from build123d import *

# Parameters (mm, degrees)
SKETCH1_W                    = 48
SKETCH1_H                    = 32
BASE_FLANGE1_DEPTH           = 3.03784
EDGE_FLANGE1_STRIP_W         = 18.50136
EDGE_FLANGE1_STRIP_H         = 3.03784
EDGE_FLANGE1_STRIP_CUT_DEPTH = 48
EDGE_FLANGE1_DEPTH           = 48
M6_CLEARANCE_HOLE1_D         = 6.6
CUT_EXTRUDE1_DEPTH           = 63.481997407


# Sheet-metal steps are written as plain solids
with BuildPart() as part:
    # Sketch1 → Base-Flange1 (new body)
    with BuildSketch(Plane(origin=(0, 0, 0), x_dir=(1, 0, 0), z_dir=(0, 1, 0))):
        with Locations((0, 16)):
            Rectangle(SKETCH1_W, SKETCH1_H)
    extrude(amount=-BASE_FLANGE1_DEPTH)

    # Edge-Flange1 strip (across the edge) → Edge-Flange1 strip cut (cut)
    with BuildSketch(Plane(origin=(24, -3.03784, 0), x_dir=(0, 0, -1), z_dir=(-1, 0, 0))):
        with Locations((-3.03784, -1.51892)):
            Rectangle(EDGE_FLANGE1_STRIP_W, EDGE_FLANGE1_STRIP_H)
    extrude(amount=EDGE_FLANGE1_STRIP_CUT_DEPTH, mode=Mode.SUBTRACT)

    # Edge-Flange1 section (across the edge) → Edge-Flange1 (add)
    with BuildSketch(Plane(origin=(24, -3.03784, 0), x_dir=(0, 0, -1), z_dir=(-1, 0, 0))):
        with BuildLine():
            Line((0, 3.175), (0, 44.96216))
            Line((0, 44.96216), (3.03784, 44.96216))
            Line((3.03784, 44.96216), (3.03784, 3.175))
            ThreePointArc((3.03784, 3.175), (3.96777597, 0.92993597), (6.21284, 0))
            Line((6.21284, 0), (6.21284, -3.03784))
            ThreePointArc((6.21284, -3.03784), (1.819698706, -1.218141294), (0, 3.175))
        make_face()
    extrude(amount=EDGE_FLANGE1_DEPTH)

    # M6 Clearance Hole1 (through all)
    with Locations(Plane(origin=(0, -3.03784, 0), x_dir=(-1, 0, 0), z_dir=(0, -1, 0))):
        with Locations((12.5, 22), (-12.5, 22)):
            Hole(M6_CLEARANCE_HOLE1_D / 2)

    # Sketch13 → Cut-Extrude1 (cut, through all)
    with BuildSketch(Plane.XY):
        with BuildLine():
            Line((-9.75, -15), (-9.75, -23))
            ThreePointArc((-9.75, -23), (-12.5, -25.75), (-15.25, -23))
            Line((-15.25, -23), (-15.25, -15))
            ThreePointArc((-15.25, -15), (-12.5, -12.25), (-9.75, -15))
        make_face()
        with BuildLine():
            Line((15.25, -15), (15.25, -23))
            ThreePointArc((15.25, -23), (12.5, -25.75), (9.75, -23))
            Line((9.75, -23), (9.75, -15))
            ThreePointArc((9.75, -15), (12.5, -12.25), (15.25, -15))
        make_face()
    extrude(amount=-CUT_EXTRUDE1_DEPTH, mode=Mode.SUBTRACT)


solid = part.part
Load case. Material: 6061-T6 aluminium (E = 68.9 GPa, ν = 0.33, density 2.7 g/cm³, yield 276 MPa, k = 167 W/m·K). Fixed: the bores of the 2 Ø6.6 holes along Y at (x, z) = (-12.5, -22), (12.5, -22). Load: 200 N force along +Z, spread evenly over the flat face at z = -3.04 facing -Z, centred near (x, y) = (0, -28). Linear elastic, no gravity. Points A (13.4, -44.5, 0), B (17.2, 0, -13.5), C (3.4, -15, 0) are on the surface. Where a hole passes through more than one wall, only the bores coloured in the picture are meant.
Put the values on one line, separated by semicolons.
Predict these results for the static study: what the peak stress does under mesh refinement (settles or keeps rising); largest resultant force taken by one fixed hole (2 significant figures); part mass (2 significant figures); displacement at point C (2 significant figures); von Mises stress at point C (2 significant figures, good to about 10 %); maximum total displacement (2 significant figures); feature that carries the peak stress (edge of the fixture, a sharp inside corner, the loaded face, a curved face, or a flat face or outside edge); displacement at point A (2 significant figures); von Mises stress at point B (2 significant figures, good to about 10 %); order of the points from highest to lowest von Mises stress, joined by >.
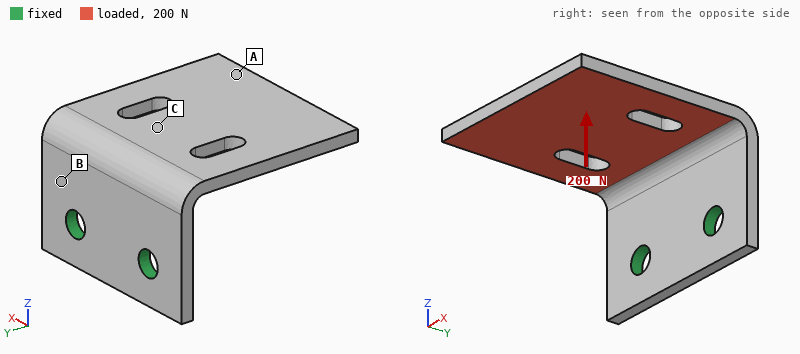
keeps rising; 100 N; 28 g; 0.24 mm; 42 MPa; 0.90 mm; edge of the fixture; 0.82 mm; 64 MPa; B > C > A
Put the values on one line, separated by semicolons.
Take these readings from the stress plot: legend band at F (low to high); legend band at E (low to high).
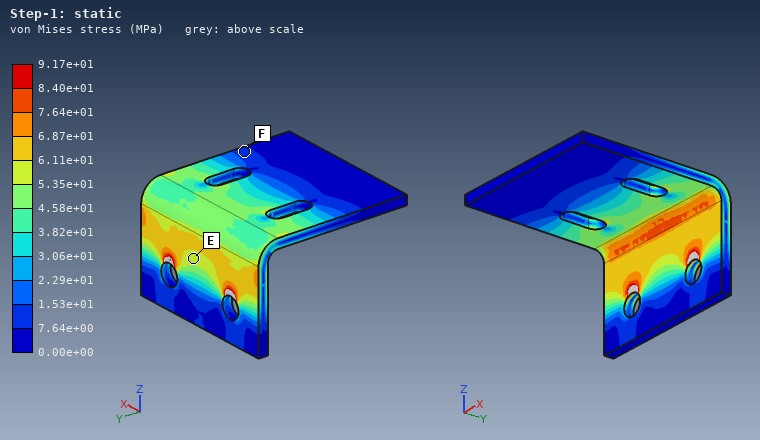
7.64e+00 to 1.53e+01 MPa; 5.35e+01 to 6.11e+01 MPa
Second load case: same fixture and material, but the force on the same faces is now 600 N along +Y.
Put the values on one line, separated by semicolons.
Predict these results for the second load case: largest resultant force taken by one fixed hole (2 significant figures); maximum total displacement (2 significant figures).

300 N; 0.46 mm
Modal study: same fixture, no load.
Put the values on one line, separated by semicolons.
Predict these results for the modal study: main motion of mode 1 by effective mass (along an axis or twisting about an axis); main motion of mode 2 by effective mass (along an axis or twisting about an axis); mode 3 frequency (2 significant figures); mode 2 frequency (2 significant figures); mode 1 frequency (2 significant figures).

along Z; along X; 2600 Hz; 1500 Hz; 730 Hz
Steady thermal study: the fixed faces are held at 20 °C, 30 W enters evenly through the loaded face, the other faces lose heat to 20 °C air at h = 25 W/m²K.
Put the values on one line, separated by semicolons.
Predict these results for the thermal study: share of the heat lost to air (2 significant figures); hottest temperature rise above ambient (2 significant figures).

12 %; 53 K
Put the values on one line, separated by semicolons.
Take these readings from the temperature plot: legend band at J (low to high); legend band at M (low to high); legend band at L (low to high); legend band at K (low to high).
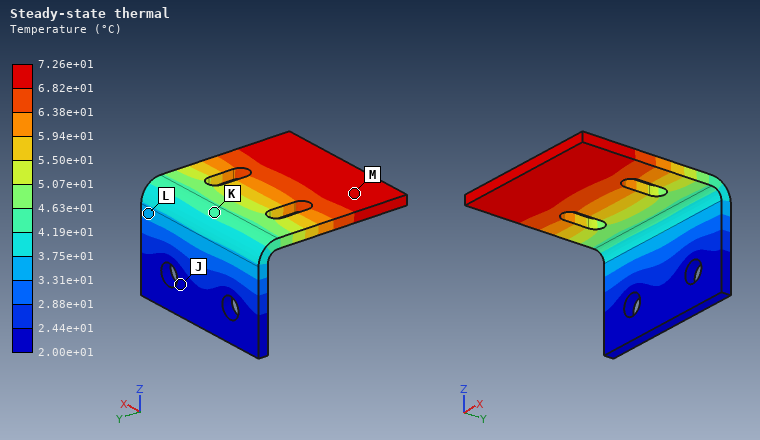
2.00e+01 to 2.44e+01 °C; 6.82e+01 to 7.26e+01 °C; 3.31e+01 to 3.75e+01 °C; 4.19e+01 to 4.63e+01 °C
